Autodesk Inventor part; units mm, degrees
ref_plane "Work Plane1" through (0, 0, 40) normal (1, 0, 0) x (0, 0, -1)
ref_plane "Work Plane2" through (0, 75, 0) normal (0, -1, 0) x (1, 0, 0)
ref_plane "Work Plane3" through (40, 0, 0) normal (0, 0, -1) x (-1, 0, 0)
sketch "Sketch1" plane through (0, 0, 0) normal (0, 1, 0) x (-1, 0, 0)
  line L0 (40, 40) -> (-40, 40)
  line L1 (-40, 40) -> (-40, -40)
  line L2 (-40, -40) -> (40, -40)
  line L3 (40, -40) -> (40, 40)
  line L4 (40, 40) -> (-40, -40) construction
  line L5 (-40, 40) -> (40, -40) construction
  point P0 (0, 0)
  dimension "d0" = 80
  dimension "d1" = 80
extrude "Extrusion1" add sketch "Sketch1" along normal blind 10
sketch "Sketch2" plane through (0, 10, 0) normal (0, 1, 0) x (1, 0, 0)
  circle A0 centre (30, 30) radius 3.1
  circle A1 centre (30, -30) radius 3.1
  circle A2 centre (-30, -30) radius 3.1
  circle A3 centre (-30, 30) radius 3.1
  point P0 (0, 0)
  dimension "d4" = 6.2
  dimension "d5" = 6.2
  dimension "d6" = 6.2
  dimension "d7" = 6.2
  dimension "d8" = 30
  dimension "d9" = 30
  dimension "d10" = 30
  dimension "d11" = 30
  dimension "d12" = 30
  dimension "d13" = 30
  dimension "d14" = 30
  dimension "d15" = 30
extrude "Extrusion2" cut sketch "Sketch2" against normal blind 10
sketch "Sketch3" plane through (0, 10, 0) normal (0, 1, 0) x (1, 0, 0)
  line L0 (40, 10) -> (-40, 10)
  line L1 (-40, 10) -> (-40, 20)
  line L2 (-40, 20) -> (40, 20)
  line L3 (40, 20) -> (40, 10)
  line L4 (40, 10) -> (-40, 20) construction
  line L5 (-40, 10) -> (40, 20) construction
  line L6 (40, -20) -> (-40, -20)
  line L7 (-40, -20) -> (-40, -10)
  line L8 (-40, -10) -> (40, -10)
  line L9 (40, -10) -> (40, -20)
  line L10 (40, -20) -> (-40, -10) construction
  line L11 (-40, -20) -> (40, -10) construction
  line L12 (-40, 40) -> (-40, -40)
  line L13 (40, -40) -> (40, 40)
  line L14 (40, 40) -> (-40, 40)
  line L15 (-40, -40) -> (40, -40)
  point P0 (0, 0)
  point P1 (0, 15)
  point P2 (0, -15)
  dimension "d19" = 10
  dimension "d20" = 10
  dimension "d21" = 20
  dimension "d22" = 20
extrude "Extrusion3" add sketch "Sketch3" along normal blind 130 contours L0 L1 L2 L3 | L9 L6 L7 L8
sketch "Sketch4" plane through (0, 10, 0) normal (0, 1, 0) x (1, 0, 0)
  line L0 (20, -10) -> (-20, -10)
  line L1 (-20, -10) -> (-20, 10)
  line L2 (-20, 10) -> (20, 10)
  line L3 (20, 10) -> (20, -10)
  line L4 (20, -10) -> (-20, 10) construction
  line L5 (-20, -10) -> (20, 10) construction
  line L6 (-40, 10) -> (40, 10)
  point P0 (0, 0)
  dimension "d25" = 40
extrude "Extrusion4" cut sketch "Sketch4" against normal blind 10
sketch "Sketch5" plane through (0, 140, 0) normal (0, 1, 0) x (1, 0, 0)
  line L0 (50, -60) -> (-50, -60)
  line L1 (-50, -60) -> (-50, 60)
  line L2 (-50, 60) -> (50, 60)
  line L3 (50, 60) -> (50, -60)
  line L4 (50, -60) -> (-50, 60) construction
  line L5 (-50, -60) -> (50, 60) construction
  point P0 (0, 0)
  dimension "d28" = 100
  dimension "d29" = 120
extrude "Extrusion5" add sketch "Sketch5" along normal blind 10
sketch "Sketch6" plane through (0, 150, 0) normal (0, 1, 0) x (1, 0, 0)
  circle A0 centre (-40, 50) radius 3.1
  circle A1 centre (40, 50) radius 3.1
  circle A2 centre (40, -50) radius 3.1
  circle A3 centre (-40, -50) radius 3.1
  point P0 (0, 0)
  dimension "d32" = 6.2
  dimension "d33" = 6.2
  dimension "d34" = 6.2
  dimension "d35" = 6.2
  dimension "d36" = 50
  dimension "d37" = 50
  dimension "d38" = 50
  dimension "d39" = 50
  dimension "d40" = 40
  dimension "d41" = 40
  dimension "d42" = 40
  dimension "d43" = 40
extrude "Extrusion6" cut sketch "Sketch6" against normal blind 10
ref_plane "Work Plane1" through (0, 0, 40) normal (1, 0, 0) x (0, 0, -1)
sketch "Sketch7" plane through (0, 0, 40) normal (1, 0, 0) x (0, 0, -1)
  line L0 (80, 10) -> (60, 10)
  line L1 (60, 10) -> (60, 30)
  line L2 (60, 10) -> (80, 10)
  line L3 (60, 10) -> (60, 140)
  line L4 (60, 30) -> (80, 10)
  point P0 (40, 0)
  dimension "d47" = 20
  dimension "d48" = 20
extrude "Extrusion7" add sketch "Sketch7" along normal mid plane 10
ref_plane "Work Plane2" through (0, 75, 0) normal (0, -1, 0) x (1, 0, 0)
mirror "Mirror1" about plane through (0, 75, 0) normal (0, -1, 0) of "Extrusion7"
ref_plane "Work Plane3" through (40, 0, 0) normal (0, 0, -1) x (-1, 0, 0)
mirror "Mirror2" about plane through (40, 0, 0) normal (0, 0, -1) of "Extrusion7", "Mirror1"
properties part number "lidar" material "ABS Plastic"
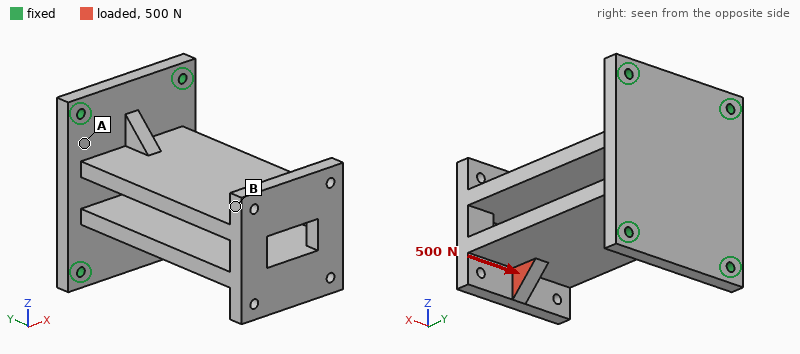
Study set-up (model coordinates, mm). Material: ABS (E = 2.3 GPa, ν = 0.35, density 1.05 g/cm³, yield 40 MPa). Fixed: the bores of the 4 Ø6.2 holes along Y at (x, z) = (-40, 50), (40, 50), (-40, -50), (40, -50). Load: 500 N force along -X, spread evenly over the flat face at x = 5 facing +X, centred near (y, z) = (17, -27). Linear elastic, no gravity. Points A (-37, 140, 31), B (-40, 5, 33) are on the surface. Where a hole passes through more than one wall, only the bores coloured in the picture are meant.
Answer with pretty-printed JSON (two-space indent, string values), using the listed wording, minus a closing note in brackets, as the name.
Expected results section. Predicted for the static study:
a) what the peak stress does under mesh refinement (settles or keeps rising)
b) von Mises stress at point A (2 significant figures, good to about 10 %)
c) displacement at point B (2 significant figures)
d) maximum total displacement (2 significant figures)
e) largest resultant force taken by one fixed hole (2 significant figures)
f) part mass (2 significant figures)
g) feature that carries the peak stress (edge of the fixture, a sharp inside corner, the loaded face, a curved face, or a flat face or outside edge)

{
  "what the peak stress does under mesh refinement": "keeps rising",
  "von Mises stress at point A": "4.6 MPa",
  "displacement at point B": "1.3 mm",
  "maximum total displacement": "2.4 mm",
  "largest resultant force taken by one fixed hole": "510 N",
  "part mass": "410 g",
  "feature that carries the peak stress": "edge of the fixture"
}
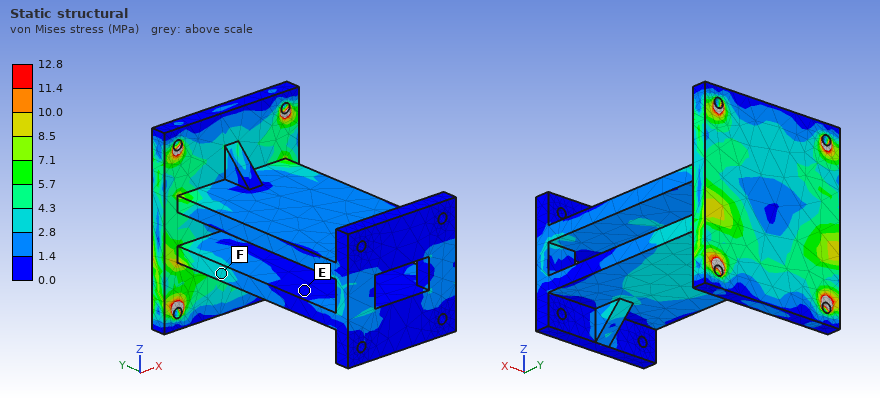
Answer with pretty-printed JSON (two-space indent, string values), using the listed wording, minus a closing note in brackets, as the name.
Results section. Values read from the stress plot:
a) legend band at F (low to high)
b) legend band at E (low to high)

{
  "legend band at F": "2.8 to 4.3 MPa",
  "legend band at E": "0.0 to 1.4 MPa"
}
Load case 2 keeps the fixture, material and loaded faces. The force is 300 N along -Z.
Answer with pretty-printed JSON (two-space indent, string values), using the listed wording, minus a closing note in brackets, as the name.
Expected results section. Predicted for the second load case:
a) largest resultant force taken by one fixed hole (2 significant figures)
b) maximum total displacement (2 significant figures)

{
  "largest resultant force taken by one fixed hole": "250 N",
  "maximum total displacement": "2.6 mm"
}
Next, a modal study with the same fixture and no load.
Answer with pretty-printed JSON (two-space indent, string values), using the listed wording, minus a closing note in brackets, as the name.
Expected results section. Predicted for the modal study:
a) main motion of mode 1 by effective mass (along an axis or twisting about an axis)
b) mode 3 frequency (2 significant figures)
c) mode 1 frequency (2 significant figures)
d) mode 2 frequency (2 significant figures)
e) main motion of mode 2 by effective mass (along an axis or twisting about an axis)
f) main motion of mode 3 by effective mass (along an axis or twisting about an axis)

{
  "main motion of mode 1 by effective mass": "along Z",
  "mode 3 frequency": "390 Hz",
  "mode 1 frequency": "150 Hz",
  "mode 2 frequency": "230 Hz",
  "main motion of mode 2 by effective mass": "along X",
  "main motion of mode 3 by effective mass": "twisting about Y"
}
